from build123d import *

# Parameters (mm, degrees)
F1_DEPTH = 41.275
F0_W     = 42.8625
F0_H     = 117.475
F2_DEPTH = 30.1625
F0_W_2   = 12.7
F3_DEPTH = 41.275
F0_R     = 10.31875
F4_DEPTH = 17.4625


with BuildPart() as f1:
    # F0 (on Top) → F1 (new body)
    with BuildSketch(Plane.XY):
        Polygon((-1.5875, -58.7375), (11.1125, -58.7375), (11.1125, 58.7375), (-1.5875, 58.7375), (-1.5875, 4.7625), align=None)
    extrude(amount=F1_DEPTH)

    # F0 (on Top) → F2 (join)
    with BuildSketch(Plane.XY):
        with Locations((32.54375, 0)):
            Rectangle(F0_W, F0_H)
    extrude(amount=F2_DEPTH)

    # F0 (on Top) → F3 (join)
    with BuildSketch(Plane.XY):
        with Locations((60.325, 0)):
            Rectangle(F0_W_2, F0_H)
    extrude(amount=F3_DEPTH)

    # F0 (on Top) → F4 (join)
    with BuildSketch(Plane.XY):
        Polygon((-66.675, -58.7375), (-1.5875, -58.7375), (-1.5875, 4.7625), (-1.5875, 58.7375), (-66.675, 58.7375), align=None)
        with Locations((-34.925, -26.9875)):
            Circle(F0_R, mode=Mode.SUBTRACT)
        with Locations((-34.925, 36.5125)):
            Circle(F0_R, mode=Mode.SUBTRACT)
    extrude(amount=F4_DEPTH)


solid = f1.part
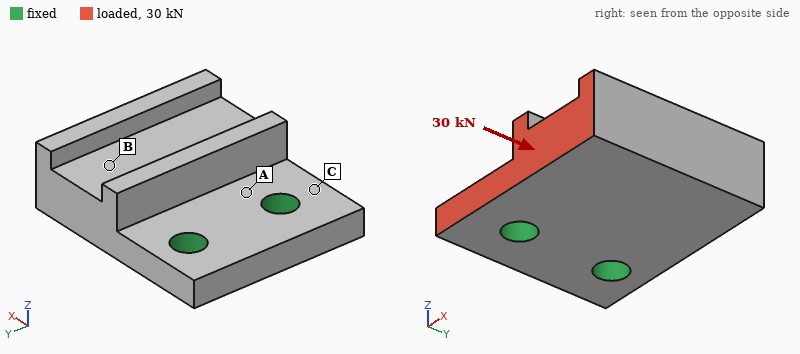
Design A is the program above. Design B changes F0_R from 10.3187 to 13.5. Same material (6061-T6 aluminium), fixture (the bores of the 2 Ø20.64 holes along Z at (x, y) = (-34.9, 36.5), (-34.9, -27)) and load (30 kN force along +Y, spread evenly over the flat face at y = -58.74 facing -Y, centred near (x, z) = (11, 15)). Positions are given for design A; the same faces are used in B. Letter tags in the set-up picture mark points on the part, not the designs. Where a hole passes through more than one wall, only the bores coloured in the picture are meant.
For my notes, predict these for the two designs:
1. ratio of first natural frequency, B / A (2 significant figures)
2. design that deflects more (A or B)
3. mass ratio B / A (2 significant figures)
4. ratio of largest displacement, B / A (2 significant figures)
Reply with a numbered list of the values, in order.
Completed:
1. 1.1
2. A
3. 0.98
4. 0.86
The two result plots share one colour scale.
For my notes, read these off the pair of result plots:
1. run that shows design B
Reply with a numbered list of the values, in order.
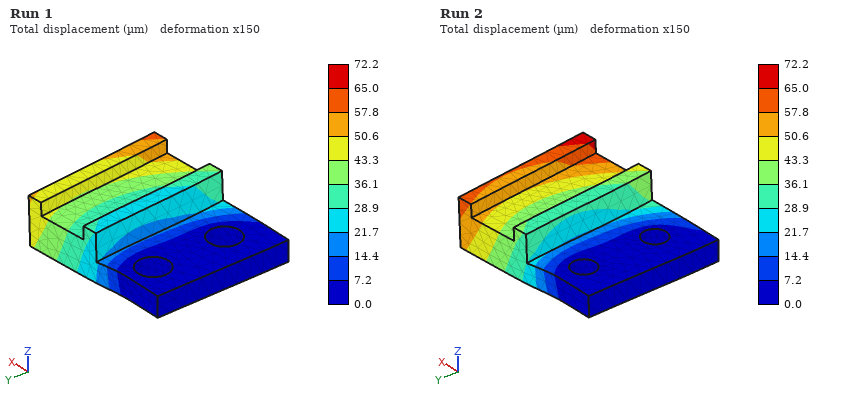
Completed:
1. Run 1
